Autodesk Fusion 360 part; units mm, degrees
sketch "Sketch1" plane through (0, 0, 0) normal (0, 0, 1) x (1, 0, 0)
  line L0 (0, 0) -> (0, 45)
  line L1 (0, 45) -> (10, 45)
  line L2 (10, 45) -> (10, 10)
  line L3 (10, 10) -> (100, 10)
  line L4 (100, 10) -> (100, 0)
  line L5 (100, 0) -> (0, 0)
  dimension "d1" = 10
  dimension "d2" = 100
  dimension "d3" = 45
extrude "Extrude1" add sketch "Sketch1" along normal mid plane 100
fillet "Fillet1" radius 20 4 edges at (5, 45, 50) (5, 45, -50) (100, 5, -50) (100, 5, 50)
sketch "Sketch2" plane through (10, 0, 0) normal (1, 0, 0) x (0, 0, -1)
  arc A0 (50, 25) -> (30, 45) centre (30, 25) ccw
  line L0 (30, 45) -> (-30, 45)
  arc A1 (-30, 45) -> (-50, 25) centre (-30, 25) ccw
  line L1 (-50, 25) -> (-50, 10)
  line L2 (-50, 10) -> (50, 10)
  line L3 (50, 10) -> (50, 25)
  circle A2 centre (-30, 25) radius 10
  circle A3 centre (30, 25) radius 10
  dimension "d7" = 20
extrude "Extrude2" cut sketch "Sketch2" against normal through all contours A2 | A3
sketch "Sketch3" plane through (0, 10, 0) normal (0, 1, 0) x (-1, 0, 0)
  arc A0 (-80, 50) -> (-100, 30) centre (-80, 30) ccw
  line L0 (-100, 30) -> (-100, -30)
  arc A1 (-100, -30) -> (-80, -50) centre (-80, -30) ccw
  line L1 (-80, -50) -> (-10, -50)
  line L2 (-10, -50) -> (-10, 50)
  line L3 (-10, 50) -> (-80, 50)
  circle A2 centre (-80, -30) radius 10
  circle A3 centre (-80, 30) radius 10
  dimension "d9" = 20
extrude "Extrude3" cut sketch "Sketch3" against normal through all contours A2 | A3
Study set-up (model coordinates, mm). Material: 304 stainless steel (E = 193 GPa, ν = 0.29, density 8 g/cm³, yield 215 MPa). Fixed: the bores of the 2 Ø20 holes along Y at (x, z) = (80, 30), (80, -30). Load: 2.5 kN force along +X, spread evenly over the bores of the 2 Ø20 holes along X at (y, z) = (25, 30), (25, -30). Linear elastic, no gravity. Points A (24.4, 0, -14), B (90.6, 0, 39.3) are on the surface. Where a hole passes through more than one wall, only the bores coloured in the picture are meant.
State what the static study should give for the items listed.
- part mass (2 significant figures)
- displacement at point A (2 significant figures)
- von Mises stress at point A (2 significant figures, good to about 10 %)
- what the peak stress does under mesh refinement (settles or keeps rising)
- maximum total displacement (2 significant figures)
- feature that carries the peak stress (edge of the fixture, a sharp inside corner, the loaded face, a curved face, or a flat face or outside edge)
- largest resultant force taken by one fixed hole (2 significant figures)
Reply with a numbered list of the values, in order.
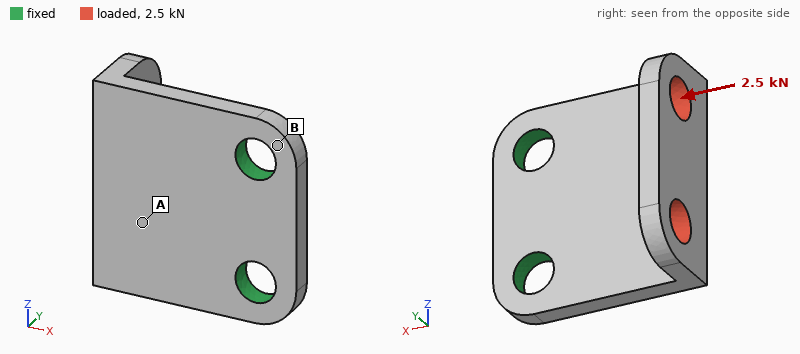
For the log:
1. 950 g
2. 0.038 mm
3. 25 MPa
4. keeps rising
5. 0.12 mm
6. edge of the fixture
7. 1.3 kN
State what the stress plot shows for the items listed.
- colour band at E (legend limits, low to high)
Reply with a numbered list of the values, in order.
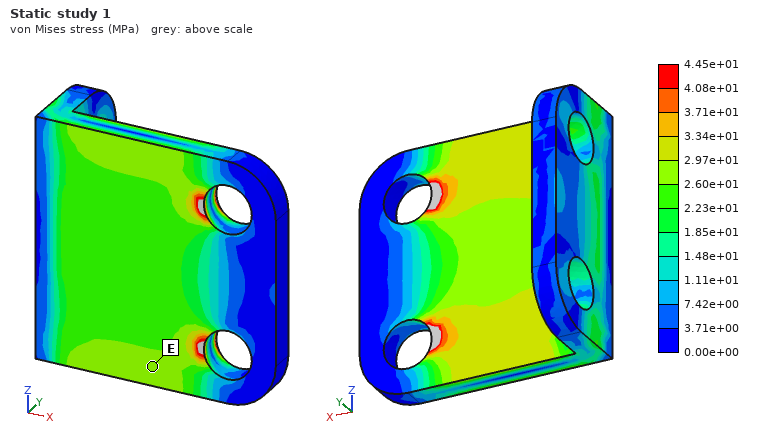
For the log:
1. 2.60e+01 to 2.97e+01 MPa
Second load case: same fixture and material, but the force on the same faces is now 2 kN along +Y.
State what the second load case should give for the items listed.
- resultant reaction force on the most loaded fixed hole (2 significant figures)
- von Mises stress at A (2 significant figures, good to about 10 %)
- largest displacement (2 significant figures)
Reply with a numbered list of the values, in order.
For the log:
1. 1.0 kN
2. 22 MPa
3. 0.19 mm
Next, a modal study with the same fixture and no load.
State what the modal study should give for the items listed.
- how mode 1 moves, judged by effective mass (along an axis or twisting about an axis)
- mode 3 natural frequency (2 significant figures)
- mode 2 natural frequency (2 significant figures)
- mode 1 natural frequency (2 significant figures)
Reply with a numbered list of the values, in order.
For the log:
1. along Y
2. 3300 Hz
3. 1800 Hz
4. 920 Hz
